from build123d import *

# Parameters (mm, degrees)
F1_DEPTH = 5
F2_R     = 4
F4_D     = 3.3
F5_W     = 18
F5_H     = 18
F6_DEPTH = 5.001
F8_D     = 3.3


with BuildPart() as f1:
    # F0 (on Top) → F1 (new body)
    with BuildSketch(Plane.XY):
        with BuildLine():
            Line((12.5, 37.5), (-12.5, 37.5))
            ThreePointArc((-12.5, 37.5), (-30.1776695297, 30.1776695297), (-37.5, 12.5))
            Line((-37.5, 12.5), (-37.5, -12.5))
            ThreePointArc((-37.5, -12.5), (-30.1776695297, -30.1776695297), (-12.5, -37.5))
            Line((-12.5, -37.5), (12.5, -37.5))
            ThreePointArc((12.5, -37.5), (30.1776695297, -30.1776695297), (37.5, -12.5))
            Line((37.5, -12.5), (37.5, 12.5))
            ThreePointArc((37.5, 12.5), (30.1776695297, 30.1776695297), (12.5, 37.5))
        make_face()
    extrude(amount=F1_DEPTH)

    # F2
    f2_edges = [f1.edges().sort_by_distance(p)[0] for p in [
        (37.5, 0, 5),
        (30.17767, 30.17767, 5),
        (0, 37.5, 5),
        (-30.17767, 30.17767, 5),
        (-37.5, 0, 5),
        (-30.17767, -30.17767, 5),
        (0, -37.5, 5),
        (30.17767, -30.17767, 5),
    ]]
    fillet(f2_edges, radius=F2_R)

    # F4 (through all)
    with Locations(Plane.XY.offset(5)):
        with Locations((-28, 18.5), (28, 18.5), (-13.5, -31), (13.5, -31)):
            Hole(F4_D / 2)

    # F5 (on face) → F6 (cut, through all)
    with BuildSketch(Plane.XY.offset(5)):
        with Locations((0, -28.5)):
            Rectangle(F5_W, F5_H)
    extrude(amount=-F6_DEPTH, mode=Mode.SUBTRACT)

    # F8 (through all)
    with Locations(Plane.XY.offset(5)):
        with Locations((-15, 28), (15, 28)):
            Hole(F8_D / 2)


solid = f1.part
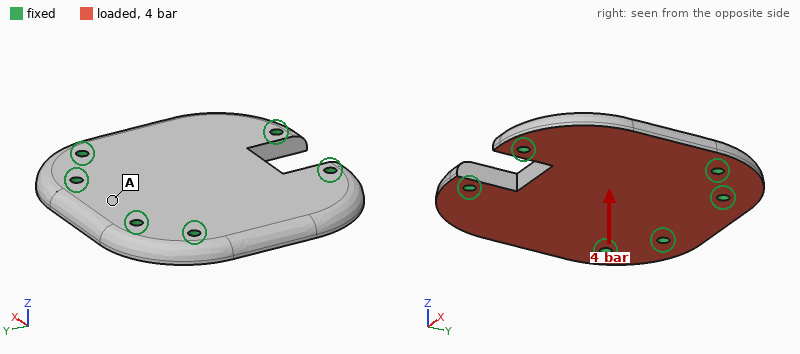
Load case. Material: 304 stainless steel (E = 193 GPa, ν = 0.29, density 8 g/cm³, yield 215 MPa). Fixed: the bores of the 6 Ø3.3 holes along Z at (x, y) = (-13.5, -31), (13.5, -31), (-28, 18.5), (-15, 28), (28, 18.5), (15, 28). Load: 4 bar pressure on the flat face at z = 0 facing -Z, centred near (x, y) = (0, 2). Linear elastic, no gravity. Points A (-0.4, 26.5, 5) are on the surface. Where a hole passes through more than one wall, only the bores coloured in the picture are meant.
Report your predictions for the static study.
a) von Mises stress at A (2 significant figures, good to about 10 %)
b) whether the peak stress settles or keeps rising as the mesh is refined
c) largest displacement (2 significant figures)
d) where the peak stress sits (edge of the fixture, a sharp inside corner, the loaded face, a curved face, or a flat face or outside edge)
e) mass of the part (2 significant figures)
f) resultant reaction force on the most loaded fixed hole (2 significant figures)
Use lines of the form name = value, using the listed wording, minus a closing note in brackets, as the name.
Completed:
von Mises stress at A = 7.9 MPa
whether the peak stress settles or keeps rising as the mesh is refined = keeps rising
largest displacement = 9.2 µm
where the peak stress sits = edge of the fixture
mass of the part = 180 g
resultant reaction force on the most loaded fixed hole = 370 N
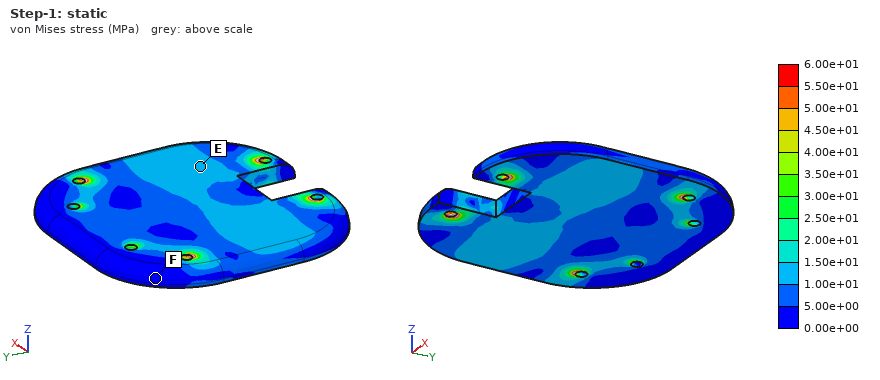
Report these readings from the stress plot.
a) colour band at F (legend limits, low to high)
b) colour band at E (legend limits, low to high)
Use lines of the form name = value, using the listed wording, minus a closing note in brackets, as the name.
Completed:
colour band at F = 0.00e+00 to 5.00e+00 MPa
colour band at E = 1.00e+01 to 1.50e+01 MPa
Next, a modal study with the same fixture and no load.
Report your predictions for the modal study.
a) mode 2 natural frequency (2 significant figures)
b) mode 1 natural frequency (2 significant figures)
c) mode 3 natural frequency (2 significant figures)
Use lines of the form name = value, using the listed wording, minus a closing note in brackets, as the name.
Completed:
mode 2 natural frequency = 7000 Hz
mode 1 natural frequency = 6800 Hz
mode 3 natural frequency = 8500 Hz
